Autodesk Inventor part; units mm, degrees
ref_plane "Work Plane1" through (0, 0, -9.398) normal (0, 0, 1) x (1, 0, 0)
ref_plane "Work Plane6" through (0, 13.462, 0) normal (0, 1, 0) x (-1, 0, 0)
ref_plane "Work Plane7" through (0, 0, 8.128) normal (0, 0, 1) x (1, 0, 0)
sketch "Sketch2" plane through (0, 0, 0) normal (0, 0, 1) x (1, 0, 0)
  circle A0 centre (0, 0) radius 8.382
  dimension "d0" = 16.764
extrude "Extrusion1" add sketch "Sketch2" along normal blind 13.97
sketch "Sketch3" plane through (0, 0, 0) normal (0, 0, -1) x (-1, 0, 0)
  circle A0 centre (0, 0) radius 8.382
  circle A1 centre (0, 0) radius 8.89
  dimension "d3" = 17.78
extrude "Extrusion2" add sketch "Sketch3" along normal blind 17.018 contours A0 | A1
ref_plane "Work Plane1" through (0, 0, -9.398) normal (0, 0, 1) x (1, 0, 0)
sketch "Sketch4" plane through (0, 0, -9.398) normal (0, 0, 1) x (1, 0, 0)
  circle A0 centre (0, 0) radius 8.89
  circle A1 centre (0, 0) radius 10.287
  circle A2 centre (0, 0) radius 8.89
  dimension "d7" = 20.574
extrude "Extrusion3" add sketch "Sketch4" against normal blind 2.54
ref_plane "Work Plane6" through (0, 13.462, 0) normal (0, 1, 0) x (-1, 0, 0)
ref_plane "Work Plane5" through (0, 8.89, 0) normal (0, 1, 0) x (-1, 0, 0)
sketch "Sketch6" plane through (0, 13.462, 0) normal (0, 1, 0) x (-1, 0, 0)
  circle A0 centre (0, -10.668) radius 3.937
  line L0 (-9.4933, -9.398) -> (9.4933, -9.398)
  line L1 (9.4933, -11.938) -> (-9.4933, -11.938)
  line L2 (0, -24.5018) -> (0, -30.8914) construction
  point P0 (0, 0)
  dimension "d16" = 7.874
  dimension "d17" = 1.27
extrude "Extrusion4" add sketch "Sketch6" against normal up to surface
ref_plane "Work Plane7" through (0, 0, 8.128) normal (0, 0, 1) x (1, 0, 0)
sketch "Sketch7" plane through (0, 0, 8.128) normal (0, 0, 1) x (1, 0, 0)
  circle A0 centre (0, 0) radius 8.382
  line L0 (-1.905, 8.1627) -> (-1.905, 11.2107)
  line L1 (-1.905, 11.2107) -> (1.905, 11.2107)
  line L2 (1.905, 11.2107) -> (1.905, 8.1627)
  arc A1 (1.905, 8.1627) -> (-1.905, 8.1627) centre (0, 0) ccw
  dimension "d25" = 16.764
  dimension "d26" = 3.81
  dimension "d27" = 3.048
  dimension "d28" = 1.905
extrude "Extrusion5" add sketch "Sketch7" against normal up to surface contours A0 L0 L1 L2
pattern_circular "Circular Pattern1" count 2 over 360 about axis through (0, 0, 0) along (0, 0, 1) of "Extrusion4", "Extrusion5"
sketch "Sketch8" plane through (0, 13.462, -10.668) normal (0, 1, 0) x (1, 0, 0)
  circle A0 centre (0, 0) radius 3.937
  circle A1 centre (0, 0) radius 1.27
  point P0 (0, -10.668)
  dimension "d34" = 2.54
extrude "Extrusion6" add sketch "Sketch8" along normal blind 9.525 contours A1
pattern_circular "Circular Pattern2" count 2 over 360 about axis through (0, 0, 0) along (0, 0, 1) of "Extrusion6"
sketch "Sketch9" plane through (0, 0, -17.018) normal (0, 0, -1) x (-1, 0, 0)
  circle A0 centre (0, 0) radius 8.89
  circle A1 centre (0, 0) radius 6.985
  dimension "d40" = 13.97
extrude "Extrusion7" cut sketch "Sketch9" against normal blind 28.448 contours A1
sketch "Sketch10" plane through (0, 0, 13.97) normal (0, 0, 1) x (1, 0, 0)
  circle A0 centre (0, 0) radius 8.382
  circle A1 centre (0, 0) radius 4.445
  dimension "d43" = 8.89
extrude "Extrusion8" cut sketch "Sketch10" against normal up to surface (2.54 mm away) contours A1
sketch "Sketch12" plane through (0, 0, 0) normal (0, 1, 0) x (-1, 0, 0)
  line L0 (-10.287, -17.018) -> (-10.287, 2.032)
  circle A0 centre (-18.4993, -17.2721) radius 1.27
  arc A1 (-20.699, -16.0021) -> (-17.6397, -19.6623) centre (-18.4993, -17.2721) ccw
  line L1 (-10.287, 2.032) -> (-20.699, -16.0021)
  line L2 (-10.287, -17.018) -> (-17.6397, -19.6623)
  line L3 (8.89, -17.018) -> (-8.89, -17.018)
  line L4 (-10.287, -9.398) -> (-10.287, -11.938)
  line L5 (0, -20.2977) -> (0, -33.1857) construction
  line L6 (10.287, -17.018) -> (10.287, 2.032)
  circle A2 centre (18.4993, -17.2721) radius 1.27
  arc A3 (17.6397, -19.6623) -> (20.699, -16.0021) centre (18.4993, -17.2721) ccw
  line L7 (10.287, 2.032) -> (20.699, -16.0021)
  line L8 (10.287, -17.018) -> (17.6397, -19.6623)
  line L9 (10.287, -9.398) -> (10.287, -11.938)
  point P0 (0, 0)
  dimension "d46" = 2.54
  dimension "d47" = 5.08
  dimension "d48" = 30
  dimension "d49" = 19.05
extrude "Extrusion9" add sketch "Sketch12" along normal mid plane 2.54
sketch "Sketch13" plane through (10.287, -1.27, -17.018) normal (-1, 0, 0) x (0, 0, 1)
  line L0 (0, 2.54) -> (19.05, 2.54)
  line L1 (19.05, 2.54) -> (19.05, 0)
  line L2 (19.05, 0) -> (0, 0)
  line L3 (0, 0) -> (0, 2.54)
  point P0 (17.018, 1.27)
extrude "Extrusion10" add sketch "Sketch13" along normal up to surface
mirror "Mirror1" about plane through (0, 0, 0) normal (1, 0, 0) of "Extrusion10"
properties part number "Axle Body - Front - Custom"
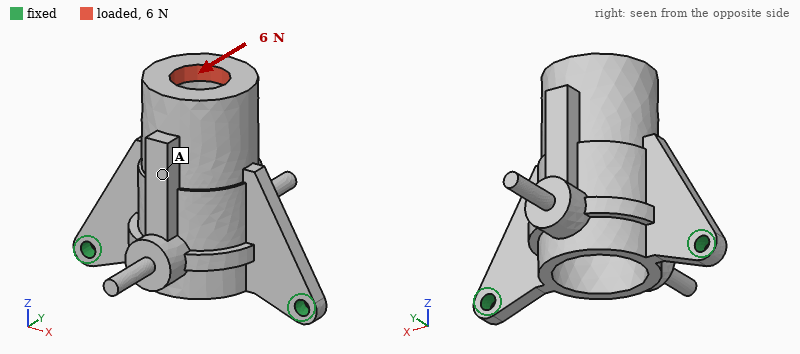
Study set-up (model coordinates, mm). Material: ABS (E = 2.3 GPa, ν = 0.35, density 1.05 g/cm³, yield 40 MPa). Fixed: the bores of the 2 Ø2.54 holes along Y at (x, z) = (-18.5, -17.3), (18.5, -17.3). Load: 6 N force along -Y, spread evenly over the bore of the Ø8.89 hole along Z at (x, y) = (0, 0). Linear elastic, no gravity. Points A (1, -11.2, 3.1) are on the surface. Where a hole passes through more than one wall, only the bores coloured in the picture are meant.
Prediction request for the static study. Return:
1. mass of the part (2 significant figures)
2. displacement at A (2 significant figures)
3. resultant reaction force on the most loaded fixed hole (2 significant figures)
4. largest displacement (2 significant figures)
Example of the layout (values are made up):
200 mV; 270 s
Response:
4.8 g; 0.49 mm; 3.0 N; 0.69 mm
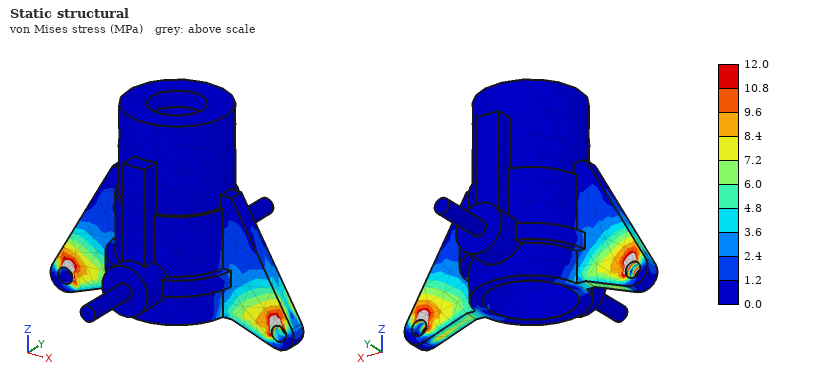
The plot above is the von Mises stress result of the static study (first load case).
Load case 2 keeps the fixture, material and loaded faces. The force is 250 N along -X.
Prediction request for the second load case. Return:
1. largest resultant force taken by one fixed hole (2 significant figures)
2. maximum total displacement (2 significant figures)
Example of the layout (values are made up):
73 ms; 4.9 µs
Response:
240 N; 0.44 mm
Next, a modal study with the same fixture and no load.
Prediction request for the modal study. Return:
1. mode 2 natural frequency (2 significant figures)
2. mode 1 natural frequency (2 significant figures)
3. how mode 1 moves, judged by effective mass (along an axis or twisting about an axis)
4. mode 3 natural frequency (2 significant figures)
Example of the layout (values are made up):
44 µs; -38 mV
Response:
2300 Hz; 400 Hz; along Y; 2400 Hz
